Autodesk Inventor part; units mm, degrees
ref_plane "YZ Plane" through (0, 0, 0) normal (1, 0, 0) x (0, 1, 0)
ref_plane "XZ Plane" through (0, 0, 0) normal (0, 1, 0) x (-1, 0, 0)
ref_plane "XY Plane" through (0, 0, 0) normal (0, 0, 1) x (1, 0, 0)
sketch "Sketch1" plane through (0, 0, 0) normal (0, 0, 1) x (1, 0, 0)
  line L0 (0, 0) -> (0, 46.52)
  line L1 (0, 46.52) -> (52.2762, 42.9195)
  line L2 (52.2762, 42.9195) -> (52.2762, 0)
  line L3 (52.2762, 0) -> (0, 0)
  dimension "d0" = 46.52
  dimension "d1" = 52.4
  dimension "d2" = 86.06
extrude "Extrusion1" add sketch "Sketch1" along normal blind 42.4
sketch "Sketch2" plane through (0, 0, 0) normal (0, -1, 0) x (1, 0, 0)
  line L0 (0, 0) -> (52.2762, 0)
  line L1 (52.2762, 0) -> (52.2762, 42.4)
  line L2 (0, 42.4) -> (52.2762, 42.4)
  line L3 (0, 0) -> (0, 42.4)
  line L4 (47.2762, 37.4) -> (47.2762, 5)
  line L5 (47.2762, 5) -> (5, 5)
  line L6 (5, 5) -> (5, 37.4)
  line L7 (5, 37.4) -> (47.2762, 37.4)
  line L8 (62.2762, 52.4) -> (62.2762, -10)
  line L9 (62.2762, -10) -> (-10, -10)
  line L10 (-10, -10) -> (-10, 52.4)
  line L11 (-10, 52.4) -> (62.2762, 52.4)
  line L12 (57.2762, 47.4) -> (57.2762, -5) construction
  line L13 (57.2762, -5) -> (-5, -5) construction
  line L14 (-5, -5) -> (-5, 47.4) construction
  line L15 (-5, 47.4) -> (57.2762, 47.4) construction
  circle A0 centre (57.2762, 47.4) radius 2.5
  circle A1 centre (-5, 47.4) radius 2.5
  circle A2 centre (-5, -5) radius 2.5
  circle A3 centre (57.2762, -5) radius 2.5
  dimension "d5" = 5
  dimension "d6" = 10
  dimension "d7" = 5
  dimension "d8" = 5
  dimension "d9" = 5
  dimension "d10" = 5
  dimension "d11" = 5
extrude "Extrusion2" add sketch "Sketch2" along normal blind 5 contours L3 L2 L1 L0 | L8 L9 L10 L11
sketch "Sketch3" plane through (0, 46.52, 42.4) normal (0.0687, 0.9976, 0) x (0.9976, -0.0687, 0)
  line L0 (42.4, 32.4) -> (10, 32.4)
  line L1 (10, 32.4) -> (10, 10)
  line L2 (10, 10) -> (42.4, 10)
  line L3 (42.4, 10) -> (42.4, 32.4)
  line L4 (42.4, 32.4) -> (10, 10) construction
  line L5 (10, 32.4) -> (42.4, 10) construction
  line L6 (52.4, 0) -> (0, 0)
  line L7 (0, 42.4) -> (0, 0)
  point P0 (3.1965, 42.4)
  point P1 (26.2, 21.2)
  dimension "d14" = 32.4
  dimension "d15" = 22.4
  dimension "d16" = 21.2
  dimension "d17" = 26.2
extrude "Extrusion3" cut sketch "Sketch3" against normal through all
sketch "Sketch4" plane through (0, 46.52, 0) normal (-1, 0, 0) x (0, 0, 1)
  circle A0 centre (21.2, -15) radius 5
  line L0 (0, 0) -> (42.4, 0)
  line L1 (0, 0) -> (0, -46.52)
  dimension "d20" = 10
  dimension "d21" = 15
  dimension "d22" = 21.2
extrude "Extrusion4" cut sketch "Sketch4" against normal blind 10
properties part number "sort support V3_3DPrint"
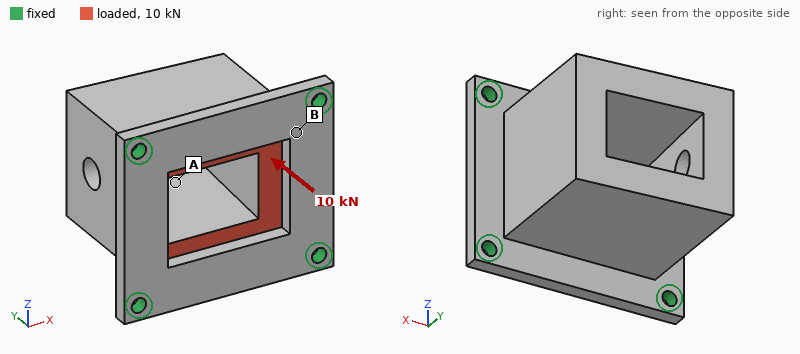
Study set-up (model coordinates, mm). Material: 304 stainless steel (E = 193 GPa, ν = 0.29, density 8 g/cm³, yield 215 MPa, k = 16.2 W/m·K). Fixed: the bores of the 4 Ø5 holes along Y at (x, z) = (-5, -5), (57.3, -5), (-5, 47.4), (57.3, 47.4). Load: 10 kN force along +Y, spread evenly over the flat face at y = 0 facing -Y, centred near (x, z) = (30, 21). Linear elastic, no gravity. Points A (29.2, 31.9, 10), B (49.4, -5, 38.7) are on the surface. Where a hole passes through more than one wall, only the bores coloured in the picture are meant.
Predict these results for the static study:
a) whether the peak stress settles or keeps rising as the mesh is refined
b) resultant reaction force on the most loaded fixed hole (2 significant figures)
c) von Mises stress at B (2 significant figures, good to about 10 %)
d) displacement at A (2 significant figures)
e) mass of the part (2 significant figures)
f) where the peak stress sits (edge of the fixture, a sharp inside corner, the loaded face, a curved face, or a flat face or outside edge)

keeps rising
3.2 kN
47 MPa
16 µm
650 g
edge of the fixture
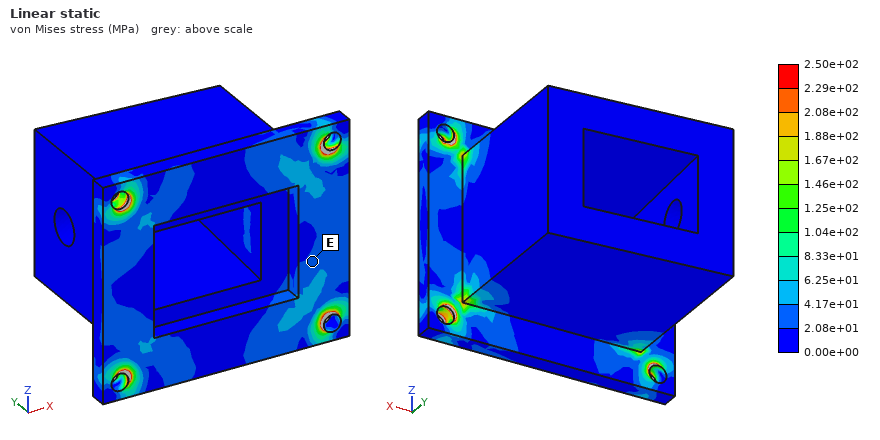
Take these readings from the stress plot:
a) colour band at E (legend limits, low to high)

2.08e+01 to 4.17e+01 MPa
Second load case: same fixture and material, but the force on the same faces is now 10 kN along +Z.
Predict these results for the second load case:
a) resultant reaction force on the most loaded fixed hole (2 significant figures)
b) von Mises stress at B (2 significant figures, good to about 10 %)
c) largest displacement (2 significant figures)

3.3 kN
26 MPa
8.5 µm
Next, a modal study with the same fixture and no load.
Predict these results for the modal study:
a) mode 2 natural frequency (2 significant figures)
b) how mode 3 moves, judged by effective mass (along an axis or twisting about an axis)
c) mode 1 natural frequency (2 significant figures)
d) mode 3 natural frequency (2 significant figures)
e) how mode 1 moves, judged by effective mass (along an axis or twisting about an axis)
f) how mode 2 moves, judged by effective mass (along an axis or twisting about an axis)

4300 Hz
along Y
3700 Hz
5100 Hz
along Z
along X
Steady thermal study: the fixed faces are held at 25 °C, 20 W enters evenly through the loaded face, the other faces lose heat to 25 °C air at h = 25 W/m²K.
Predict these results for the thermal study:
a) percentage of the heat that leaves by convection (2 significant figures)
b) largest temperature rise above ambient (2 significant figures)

52 %
38 K
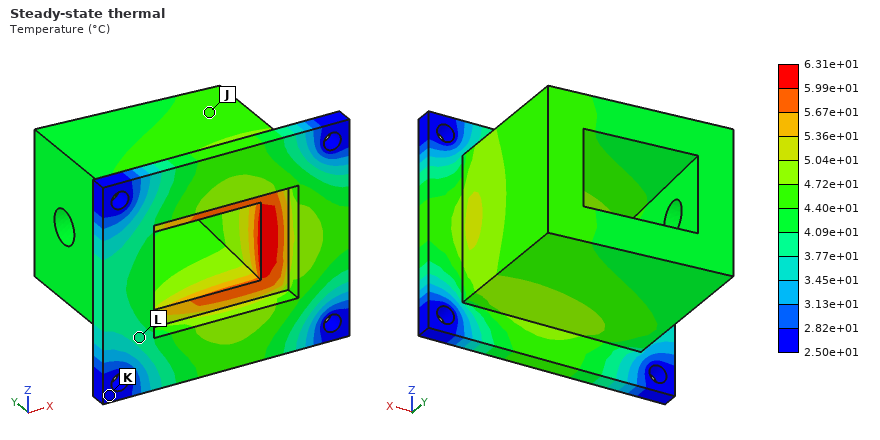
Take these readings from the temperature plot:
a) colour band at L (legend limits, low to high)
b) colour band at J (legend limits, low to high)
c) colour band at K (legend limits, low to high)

3.77e+01 to 4.09e+01 °C
4.40e+01 to 4.72e+01 °C
2.50e+01 to 2.82e+01 °C
